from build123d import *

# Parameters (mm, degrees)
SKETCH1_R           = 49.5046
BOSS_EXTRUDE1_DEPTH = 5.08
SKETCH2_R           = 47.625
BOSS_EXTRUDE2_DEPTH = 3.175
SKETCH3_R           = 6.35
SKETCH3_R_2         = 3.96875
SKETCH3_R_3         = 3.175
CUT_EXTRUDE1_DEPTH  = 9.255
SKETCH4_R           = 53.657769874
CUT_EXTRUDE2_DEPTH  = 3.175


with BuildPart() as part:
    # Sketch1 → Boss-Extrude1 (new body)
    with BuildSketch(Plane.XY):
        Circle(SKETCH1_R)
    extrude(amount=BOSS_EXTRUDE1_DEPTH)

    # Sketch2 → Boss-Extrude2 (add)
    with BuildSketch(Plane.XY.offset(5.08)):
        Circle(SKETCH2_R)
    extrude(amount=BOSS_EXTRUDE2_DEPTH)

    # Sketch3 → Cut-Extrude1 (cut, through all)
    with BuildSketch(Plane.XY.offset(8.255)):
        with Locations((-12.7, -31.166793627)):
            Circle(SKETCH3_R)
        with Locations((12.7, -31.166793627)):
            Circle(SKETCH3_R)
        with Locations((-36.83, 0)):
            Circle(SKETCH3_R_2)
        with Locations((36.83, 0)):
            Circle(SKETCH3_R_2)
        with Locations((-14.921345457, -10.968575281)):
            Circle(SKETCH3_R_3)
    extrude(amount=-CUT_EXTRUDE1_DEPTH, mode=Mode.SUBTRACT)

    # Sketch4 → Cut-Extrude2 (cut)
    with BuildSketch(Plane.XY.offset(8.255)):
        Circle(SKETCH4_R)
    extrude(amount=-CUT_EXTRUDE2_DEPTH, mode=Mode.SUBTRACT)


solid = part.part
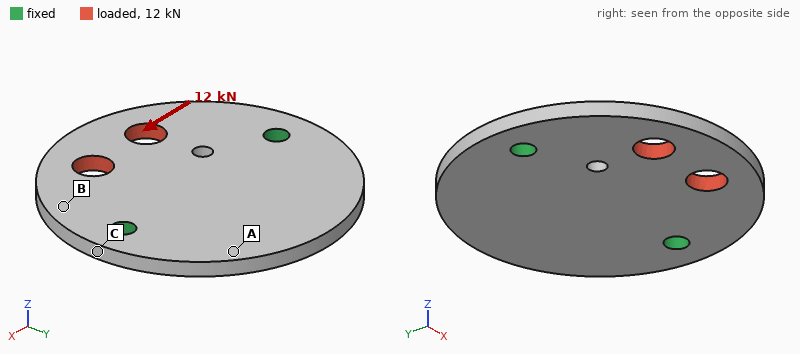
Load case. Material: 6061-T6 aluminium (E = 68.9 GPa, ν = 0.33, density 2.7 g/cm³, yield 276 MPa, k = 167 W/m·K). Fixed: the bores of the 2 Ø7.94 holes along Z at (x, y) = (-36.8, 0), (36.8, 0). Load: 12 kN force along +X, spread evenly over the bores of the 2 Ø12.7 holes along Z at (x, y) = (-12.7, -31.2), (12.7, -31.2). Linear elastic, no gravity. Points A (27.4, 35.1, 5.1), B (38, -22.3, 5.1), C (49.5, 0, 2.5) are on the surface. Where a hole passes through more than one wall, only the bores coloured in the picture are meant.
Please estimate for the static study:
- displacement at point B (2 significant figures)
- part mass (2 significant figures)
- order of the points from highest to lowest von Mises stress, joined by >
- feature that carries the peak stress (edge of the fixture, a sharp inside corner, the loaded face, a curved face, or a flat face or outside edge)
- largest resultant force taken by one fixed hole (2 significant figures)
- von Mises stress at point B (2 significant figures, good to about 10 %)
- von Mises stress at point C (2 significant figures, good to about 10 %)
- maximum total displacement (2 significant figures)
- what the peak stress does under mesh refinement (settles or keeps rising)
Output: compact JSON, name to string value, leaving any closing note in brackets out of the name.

{"displacement at point B": "32 µm", "part mass": "100 g", "order of the points from highest to lowest von Mises stress, joined by >": "C > B > A", "feature that carries the peak stress": "edge of the fixture", "largest resultant force taken by one fixed hole": "7.8 kN", "von Mises stress at point B": "32 MPa", "von Mises stress at point C": "51 MPa", "maximum total displacement": "64 µm", "what the peak stress does under mesh refinement": "keeps rising"}
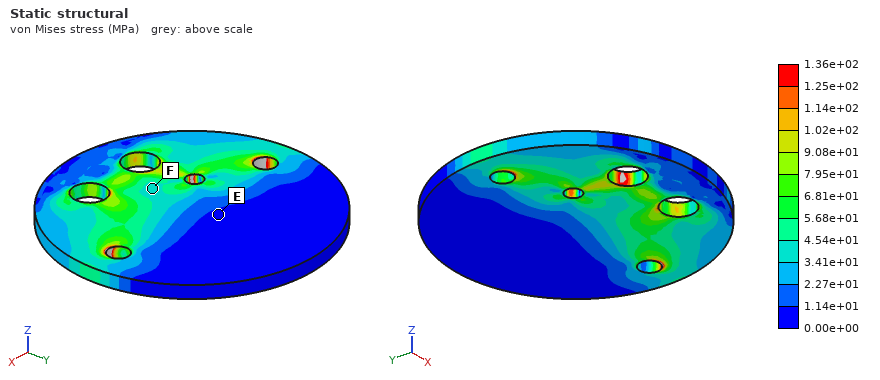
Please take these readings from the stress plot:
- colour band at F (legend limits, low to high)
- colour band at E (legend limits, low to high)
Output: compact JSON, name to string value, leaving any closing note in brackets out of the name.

{"colour band at F": "3.41e+01 to 4.54e+01 MPa", "colour band at E": "0.00e+00 to 1.14e+01 MPa"}
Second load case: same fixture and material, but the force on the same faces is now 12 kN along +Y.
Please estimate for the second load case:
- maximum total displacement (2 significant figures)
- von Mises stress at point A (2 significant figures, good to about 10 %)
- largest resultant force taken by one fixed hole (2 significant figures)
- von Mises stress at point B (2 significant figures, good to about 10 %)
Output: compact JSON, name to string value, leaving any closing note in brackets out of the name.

{"maximum total displacement": "38 µm", "von Mises stress at point A": "12 MPa", "largest resultant force taken by one fixed hole": "6.1 kN", "von Mises stress at point B": "18 MPa"}
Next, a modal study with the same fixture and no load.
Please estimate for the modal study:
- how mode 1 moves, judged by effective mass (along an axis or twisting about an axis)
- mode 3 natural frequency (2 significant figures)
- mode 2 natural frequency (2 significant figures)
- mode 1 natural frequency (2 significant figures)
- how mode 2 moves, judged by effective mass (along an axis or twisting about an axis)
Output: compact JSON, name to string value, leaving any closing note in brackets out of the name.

{"how mode 1 moves, judged by effective mass": "twisting about X", "mode 3 natural frequency": "4500 Hz", "mode 2 natural frequency": "2200 Hz", "mode 1 natural frequency": "1700 Hz", "how mode 2 moves, judged by effective mass": "along Z"}
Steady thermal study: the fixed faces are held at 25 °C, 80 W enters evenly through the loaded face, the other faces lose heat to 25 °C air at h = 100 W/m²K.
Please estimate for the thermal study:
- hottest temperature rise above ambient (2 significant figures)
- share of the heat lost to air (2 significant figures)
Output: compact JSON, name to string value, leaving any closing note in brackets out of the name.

{"hottest temperature rise above ambient": "49 K", "share of the heat lost to air": "30 %"}
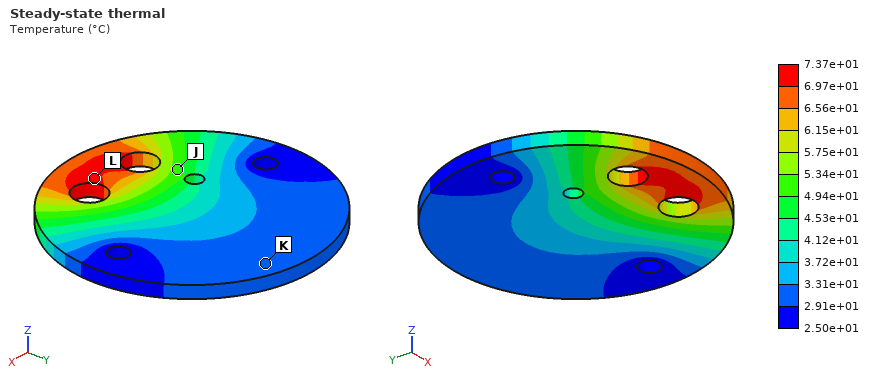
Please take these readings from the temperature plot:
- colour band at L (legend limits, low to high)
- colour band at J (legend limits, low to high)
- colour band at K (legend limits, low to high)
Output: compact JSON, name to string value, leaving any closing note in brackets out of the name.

{"colour band at L": "6.97e+01 to 7.37e+01 °C", "colour band at J": "4.94e+01 to 5.34e+01 °C", "colour band at K": "2.91e+01 to 3.31e+01 °C"}
